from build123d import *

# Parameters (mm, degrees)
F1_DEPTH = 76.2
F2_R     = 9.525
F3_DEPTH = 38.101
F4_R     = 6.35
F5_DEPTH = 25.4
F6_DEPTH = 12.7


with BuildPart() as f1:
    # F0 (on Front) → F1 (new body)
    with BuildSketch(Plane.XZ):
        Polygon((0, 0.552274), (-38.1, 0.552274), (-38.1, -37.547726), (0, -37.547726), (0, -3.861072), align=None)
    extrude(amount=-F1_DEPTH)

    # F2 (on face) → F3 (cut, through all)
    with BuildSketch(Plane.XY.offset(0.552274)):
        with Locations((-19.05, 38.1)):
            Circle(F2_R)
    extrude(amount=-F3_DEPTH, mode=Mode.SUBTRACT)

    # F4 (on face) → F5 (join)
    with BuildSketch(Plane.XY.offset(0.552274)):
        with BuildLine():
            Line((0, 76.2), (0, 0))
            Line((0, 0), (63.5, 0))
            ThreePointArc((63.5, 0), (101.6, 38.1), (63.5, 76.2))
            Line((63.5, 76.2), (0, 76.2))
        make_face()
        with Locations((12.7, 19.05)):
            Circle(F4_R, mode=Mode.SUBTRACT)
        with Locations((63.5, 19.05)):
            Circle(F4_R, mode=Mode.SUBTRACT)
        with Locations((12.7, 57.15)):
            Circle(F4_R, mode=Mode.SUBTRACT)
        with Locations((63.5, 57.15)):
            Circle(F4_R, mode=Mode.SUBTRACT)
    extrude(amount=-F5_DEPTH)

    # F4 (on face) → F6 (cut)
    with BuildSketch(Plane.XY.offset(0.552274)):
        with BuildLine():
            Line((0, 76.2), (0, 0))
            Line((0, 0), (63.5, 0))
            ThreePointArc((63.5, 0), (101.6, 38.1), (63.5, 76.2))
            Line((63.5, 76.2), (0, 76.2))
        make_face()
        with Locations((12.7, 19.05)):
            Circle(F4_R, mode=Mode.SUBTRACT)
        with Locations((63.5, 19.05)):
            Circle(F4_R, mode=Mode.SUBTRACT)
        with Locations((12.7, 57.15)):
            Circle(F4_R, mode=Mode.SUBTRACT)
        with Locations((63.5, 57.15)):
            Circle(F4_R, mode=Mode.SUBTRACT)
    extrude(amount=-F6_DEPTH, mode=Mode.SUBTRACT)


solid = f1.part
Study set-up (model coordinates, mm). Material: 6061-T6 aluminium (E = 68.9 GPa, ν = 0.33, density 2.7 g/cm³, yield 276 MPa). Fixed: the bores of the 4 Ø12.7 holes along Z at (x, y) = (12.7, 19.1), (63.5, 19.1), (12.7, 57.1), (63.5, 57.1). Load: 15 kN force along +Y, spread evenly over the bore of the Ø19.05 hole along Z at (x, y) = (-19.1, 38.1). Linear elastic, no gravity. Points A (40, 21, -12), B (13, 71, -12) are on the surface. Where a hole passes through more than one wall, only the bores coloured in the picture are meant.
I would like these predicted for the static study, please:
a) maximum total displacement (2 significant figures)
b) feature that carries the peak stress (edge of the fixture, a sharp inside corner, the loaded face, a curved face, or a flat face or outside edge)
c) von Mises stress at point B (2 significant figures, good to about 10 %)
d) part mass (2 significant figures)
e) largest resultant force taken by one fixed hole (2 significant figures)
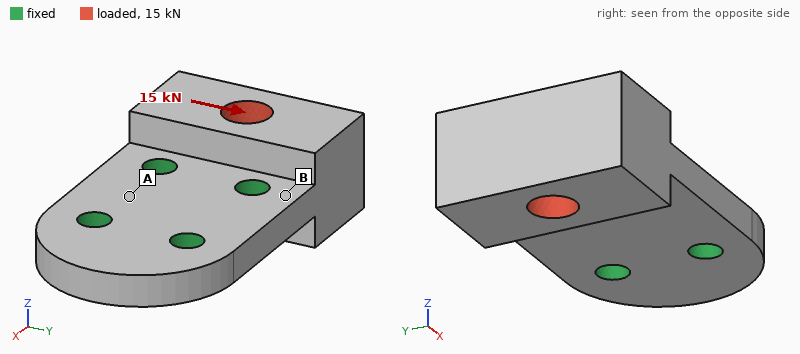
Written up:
34 µm
edge of the fixture
20 MPa
500 g
11 kN
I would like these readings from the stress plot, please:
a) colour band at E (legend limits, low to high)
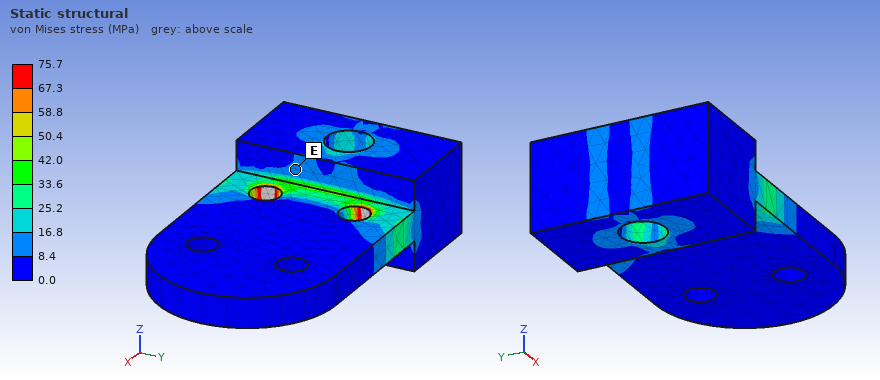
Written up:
8.4 to 16.8 MPa
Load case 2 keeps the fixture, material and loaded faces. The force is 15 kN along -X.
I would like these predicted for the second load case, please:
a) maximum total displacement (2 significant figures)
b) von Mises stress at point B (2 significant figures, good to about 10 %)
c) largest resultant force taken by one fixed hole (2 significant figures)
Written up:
11 µm
6.2 MPa
7.2 kN
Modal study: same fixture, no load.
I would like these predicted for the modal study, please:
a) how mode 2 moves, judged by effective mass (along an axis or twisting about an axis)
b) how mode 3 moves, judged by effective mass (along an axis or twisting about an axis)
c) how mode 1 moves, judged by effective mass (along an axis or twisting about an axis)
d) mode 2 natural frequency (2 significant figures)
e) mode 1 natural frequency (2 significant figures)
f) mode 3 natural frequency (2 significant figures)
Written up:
twisting about X
along Y
along Z
6500 Hz
2700 Hz
7300 Hz
